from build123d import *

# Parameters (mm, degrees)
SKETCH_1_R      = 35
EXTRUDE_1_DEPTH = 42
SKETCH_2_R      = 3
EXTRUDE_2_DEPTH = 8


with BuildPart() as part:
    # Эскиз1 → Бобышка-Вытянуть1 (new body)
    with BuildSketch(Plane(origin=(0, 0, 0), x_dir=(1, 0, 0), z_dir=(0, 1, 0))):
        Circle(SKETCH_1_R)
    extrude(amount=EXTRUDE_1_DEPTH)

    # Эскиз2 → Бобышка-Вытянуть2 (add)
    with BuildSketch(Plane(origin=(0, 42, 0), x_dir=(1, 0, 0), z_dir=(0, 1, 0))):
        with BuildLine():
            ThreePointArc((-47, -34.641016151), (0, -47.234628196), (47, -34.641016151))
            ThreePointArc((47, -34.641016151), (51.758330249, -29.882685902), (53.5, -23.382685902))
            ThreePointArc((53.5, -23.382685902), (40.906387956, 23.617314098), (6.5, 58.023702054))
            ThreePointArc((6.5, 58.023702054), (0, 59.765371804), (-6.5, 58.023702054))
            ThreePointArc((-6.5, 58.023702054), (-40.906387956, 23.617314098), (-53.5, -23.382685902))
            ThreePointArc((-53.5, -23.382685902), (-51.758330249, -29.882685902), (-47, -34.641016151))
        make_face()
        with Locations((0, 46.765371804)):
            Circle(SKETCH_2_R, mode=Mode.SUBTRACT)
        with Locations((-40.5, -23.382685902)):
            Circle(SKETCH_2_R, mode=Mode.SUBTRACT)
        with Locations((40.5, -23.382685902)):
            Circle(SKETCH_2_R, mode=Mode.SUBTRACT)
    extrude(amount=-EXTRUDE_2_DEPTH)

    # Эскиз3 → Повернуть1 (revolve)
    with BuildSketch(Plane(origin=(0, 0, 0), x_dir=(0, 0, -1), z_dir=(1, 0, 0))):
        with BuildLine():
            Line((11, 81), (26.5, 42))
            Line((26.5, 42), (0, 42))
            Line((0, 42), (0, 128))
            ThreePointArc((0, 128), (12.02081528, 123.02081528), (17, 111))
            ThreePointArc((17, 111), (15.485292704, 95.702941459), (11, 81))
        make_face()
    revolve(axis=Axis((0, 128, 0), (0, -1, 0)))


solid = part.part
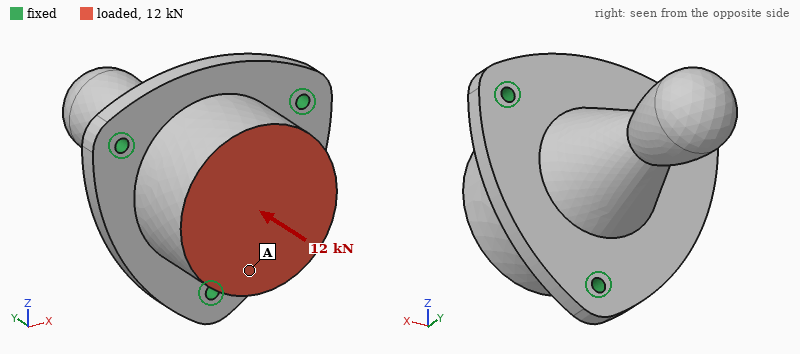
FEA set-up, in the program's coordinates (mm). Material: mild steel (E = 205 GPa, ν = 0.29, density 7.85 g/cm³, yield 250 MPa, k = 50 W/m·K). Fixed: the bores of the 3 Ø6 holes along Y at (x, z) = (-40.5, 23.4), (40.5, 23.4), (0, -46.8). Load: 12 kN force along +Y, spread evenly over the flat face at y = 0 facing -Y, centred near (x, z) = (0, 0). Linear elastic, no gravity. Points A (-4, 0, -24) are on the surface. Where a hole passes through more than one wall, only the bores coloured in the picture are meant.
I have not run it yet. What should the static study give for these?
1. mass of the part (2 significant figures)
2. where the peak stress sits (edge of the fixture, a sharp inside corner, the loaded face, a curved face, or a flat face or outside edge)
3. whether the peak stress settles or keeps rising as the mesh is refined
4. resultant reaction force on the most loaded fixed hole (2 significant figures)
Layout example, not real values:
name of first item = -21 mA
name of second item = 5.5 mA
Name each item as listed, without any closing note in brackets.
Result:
mass of the part = 2.2 kg
where the peak stress sits = edge of the fixture
whether the peak stress settles or keeps rising as the mesh is refined = keeps rising
resultant reaction force on the most loaded fixed hole = 4.2 kN
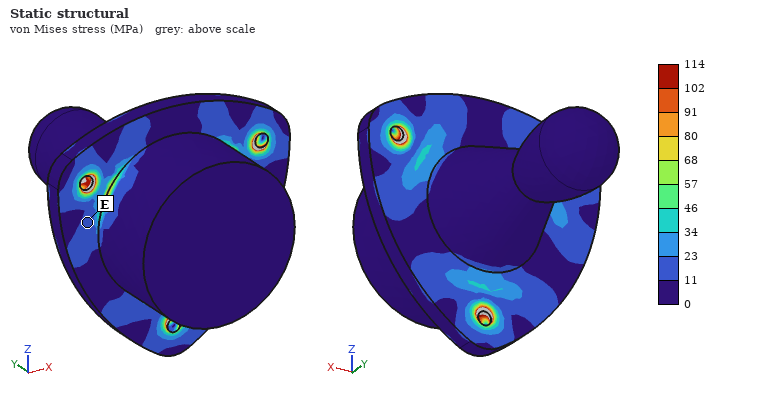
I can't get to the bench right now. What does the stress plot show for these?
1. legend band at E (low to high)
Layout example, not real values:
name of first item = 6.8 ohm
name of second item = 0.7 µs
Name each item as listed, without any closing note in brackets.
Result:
legend band at E = 11 to 23 MPa
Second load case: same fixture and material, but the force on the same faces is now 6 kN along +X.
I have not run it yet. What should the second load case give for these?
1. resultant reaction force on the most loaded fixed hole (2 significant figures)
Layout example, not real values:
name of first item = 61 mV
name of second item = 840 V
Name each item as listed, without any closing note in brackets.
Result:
resultant reaction force on the most loaded fixed hole = 4.0 kN
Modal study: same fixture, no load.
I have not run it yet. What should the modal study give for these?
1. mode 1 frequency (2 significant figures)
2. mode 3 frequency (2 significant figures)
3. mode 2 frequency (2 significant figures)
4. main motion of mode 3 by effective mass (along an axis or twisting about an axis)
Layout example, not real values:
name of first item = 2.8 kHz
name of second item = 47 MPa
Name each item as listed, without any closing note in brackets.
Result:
mode 1 frequency = 2500 Hz
mode 3 frequency = 3800 Hz
mode 2 frequency = 2500 Hz
main motion of mode 3 by effective mass = along Y
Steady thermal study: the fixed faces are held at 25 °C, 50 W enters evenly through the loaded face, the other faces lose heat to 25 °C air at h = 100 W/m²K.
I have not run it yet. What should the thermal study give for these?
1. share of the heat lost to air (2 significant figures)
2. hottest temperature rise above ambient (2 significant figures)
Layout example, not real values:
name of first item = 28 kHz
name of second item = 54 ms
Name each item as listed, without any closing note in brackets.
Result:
share of the heat lost to air = 55 %
hottest temperature rise above ambient = 19 K
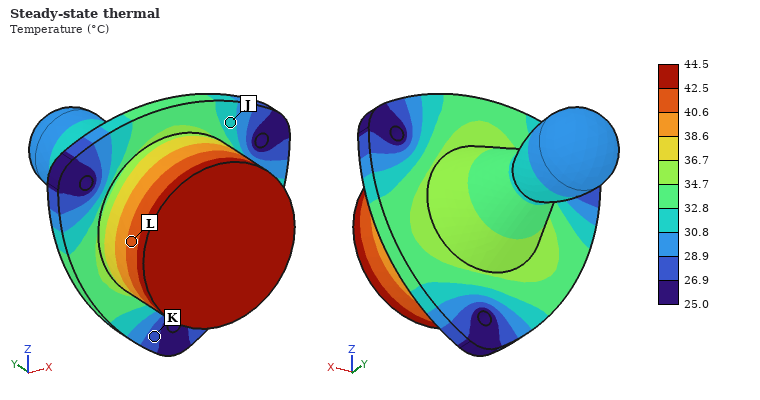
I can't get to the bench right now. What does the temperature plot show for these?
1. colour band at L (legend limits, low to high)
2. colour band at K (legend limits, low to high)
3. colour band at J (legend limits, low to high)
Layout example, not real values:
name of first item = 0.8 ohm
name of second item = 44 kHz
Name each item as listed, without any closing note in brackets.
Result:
colour band at L = 40.6 to 42.5 °C
colour band at K = 26.9 to 28.9 °C
colour band at J = 30.8 to 32.8 °C
